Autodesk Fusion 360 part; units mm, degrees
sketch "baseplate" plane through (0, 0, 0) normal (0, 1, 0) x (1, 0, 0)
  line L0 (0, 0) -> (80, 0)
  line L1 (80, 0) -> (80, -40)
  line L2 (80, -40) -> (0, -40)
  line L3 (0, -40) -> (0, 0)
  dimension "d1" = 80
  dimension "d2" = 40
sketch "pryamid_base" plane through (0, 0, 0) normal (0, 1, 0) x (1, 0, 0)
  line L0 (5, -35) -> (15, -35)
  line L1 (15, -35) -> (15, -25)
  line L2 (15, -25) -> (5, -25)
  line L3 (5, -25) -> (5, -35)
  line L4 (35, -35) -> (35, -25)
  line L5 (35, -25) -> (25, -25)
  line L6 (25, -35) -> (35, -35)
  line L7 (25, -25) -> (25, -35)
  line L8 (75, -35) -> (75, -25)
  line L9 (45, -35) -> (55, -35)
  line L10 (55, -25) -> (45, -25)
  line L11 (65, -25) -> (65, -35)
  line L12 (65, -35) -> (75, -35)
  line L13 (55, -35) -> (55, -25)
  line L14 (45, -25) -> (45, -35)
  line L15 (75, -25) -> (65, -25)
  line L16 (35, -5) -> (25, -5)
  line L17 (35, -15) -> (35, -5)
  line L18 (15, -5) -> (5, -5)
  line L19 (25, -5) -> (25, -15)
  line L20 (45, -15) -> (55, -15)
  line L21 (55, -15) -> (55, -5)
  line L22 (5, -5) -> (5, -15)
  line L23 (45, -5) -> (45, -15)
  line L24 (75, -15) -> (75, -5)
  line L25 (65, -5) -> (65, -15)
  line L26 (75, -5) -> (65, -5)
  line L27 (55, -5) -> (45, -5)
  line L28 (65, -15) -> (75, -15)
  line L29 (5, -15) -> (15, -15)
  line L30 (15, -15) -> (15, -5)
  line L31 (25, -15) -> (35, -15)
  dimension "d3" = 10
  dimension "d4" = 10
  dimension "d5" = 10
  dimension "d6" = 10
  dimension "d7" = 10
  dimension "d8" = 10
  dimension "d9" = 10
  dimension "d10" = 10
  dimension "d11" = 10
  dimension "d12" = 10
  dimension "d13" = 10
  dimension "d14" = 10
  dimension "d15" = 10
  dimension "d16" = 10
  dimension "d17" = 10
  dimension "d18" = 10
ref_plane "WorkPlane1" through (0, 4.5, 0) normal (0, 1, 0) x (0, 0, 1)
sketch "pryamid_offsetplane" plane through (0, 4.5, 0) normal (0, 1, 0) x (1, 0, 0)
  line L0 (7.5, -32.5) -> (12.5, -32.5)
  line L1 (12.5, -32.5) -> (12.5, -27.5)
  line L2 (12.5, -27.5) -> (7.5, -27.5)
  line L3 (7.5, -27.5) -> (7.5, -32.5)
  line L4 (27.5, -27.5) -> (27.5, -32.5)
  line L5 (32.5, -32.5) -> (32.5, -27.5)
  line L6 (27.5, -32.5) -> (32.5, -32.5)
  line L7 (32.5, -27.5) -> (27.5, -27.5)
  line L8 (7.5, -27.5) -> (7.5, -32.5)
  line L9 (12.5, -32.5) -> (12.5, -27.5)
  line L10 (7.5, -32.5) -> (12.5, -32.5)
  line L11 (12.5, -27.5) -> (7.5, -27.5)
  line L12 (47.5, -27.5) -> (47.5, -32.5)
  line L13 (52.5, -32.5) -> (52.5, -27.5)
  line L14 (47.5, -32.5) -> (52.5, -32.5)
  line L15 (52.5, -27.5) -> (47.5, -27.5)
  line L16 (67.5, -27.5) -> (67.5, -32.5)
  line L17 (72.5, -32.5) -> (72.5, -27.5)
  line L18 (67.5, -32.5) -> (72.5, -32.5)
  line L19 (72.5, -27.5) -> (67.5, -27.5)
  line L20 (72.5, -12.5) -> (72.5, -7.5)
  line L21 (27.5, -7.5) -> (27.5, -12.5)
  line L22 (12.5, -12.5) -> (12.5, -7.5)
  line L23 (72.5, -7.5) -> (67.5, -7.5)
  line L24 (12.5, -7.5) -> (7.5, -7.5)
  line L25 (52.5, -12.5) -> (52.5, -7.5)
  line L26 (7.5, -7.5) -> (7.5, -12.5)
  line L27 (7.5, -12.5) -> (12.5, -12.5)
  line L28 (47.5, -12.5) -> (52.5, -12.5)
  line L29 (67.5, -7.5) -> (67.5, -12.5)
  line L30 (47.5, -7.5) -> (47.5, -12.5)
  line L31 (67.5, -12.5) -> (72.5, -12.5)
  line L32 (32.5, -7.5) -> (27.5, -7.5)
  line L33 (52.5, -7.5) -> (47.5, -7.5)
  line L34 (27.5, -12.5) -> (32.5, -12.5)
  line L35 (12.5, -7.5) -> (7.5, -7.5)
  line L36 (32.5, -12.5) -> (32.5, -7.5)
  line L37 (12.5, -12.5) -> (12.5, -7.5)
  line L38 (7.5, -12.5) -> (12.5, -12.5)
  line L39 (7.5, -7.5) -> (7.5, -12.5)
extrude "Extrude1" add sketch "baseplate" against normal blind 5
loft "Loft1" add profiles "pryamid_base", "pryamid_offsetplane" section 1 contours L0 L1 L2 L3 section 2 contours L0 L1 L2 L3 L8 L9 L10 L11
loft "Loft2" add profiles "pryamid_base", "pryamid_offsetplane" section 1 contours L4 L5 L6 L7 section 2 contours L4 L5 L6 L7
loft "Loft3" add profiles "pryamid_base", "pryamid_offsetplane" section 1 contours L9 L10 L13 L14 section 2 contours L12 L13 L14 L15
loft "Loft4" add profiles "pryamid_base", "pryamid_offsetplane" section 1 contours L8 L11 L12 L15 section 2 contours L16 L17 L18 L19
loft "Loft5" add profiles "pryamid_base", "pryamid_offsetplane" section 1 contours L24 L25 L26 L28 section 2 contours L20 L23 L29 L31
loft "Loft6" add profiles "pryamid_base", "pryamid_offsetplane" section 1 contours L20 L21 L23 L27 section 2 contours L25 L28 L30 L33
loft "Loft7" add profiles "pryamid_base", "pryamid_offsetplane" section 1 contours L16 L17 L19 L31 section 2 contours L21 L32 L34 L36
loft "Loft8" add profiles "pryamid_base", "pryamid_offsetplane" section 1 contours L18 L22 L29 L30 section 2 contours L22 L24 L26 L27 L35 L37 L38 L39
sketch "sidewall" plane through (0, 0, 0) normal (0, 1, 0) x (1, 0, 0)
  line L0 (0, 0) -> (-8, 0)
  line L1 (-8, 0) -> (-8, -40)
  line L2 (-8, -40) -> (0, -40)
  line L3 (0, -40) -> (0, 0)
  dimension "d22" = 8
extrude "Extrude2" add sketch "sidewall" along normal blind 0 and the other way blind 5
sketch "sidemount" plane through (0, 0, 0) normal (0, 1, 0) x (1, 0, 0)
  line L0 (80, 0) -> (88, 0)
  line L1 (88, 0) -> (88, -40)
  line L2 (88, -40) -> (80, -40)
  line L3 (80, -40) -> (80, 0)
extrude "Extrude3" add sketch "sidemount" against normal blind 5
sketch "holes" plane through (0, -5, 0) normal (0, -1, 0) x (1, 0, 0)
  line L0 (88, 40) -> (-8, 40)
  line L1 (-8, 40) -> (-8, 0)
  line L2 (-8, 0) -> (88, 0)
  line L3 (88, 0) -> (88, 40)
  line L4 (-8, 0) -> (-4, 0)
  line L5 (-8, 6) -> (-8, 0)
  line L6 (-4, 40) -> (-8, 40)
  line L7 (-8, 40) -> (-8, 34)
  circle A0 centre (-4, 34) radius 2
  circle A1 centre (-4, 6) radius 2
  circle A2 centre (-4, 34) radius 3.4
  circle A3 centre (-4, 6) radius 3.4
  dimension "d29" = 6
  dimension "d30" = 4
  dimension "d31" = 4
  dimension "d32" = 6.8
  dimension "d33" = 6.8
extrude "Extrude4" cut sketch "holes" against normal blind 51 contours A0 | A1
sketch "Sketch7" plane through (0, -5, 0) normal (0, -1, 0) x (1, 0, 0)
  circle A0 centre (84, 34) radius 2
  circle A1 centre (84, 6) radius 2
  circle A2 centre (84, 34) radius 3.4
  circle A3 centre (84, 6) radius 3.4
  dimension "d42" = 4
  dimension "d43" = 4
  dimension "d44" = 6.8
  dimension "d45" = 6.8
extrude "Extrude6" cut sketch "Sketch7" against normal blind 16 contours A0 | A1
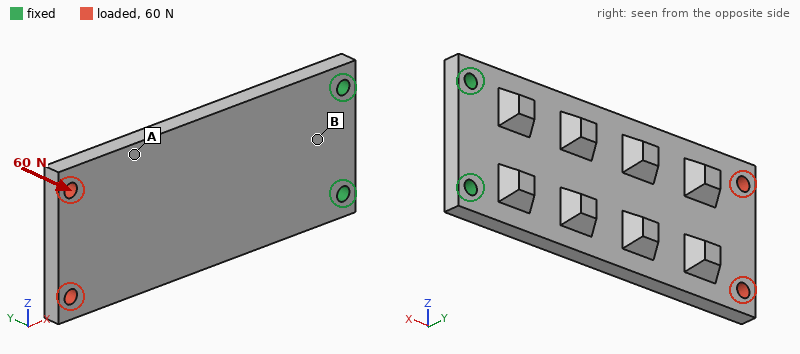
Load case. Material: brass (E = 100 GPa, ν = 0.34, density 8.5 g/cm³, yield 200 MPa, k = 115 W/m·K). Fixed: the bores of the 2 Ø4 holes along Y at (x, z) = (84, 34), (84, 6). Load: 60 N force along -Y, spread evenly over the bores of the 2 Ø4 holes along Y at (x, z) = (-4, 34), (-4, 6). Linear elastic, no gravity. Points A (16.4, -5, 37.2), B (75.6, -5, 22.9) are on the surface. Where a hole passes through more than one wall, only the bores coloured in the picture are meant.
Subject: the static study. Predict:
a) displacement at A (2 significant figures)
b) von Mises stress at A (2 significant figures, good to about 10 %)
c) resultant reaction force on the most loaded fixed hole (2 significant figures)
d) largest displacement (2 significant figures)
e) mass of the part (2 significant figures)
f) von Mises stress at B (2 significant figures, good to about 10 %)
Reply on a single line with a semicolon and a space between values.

0.20 mm; 7.0 MPa; 30 N; 0.32 mm; 180 g; 21 MPa
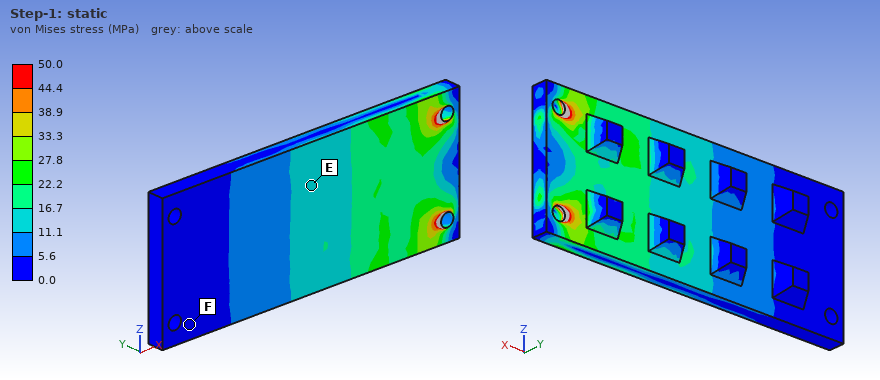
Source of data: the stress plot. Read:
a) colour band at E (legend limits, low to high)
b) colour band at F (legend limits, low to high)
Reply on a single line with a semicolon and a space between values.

11.1 to 16.7 MPa; 0.0 to 5.6 MPa
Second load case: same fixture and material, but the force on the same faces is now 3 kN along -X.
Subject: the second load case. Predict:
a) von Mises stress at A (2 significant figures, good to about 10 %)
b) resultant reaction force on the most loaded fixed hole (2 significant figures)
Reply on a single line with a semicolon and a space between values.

19 MPa; 1.5 kN
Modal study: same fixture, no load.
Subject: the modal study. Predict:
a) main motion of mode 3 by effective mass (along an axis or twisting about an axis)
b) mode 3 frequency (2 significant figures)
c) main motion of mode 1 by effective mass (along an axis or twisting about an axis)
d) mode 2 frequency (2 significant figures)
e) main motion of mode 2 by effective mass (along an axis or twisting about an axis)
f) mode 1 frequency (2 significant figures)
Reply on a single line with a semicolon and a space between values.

along Y; 2100 Hz; along Y; 1700 Hz; twisting about X; 330 Hz
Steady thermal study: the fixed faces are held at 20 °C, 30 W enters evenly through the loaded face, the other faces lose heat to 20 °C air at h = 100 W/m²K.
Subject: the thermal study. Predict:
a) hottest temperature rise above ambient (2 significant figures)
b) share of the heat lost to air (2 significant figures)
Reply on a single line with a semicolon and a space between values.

61 K; 71 %
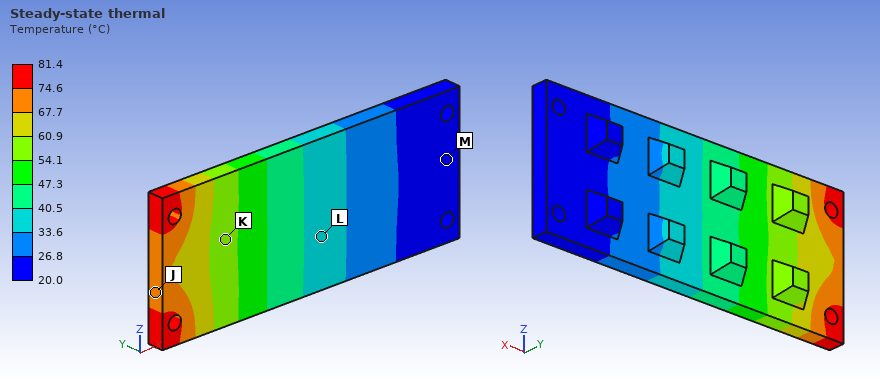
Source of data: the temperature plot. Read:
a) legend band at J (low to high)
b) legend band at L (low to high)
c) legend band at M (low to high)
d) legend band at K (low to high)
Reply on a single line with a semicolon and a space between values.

67.7 to 74.6 °C; 33.6 to 40.5 °C; 20.0 to 26.8 °C; 54.1 to 60.9 °C
